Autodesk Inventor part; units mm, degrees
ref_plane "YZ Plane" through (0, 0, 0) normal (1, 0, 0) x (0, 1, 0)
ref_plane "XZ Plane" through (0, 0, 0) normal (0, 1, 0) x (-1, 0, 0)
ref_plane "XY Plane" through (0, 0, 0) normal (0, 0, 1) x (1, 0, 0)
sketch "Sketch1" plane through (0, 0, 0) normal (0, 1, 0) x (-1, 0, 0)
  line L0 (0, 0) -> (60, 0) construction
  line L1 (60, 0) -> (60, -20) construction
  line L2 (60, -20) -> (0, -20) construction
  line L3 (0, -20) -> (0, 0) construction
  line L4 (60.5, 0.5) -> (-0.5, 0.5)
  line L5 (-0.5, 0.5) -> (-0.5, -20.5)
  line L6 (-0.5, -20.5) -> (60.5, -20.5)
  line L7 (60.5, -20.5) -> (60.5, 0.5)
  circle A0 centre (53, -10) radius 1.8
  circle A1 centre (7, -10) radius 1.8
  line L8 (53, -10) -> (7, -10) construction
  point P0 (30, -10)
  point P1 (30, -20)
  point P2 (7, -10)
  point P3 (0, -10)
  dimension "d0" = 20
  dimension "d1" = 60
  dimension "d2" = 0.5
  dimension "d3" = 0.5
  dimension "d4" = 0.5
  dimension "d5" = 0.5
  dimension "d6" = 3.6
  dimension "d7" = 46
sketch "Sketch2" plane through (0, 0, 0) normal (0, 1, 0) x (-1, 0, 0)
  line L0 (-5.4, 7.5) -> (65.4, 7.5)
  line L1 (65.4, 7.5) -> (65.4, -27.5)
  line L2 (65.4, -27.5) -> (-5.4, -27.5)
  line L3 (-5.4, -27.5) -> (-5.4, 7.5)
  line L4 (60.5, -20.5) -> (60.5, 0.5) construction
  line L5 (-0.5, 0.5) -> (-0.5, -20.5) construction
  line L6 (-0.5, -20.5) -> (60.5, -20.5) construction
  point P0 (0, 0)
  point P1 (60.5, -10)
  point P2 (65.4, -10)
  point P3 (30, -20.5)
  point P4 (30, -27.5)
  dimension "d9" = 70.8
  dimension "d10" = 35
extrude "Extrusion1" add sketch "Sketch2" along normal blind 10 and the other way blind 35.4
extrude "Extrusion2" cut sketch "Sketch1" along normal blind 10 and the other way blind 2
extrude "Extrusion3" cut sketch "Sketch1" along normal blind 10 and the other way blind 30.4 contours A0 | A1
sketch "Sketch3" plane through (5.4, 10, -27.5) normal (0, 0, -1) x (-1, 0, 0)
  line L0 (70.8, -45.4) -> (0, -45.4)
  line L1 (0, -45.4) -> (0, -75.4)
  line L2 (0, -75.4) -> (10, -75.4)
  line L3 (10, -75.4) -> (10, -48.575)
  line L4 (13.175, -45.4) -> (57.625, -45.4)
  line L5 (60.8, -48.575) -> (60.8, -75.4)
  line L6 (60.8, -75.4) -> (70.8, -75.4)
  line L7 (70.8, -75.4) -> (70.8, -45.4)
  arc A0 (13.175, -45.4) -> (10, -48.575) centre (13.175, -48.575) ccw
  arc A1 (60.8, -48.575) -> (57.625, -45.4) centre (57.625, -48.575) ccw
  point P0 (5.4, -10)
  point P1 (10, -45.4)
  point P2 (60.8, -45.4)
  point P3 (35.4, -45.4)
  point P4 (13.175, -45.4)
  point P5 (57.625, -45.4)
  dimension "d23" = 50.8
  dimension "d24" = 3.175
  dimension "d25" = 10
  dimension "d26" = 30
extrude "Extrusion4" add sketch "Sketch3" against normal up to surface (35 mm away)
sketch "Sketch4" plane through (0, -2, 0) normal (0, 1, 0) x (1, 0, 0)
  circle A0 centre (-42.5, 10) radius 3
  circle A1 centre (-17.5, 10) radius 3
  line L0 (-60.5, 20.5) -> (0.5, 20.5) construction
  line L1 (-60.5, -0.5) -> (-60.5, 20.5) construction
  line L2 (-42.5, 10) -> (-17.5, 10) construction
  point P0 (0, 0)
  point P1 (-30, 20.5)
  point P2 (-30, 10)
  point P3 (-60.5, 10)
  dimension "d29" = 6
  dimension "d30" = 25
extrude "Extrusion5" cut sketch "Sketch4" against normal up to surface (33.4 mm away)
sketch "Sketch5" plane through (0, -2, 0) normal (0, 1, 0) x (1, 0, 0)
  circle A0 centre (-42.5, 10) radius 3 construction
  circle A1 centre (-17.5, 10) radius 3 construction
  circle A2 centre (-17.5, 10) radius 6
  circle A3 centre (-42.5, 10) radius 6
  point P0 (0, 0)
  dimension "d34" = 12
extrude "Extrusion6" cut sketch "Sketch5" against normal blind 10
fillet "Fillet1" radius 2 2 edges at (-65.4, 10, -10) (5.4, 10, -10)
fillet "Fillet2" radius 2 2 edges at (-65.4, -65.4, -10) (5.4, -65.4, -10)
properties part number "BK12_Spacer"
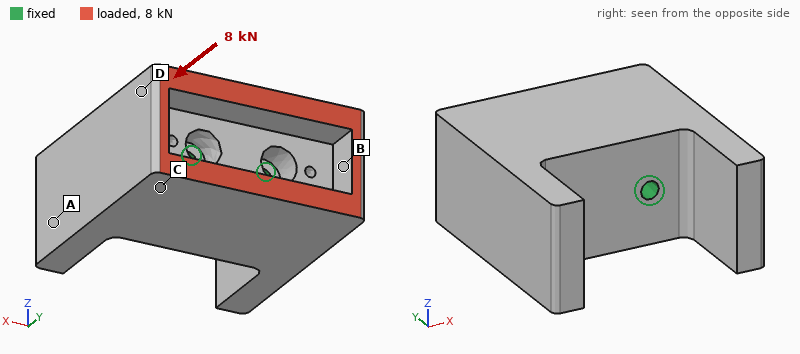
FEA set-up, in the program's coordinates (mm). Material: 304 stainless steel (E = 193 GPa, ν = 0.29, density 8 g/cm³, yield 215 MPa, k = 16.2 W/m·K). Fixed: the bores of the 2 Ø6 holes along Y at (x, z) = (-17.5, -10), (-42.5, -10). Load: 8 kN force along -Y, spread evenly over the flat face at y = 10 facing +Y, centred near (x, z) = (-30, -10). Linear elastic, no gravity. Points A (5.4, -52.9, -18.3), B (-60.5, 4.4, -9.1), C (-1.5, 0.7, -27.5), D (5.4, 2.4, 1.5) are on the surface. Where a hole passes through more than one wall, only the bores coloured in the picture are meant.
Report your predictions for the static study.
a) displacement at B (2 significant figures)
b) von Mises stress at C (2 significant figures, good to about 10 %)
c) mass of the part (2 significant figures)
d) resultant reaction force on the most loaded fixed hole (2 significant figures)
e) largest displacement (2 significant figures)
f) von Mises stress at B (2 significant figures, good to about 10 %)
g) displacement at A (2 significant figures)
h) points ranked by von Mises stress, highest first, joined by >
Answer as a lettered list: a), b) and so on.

a) 1.6 µm
b) 6.7 MPa
c) 910 g
d) 4.0 kN
e) 2.1 µm
f) 9.3 MPa
g) 1.5 µm
h) B > C > D > A
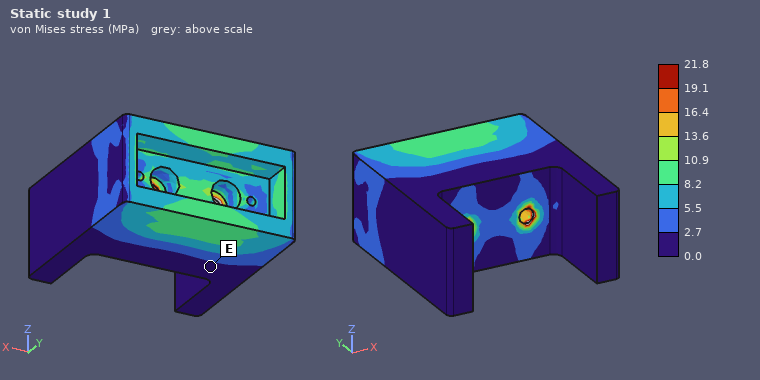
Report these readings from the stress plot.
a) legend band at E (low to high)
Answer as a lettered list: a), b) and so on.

a) 0.0 to 2.7 MPa
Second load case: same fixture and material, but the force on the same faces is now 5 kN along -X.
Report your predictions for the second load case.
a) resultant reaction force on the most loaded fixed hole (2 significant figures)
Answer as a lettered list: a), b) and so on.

a) 4.4 kN
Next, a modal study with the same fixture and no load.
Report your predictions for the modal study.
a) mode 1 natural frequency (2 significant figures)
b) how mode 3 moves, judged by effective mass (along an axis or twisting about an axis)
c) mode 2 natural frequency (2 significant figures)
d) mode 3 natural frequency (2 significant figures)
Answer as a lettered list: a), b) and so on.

a) 5900 Hz
b) twisting about X
c) 6200 Hz
d) 7600 Hz
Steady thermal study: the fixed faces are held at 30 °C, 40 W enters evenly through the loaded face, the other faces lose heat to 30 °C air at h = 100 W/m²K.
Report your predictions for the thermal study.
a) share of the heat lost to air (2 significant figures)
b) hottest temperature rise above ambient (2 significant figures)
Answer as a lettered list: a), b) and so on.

a) 56 %
b) 43 K
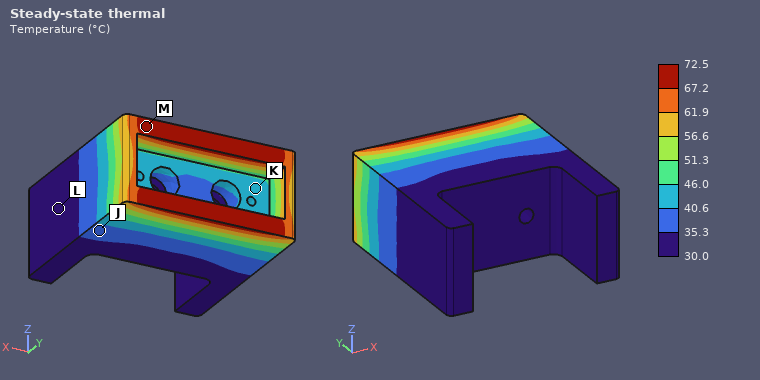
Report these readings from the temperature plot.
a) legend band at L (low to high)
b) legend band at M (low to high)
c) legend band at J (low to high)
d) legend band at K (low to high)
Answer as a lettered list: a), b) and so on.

a) 30.0 to 35.3 °C
b) 67.2 to 72.5 °C
c) 35.3 to 40.6 °C
d) 40.6 to 46.0 °C
